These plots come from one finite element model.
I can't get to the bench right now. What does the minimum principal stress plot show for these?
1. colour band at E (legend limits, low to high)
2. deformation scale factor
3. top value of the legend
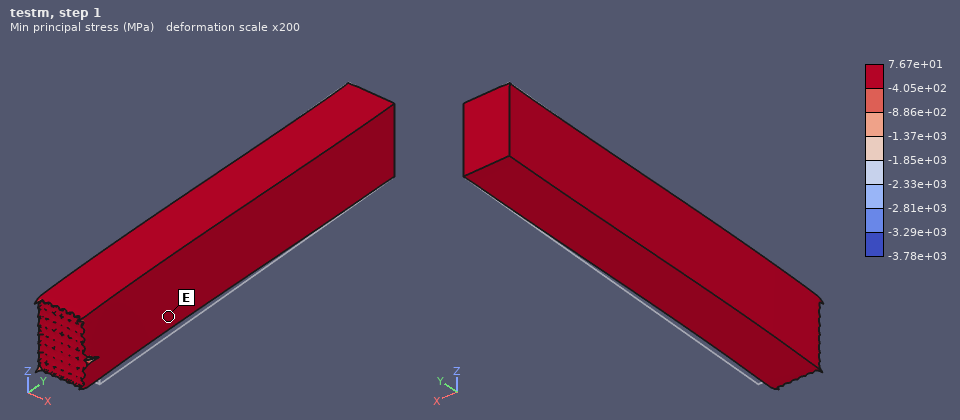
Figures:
-4.05e+02 to 7.67e+01 MPa
200
7.67e+01 MPa
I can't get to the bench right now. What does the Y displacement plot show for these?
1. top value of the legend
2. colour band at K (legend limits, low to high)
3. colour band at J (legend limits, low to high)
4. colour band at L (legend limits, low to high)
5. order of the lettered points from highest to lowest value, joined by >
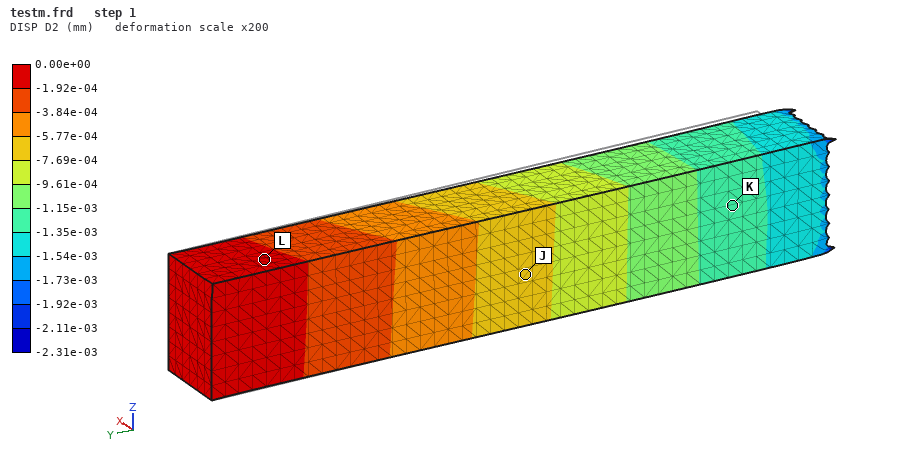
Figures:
0.00e+00 mm
-1.35e-03 to -1.15e-03 mm
-7.69e-04 to -5.77e-04 mm
-1.92e-04 to 0.00e+00 mm
L > J > K
